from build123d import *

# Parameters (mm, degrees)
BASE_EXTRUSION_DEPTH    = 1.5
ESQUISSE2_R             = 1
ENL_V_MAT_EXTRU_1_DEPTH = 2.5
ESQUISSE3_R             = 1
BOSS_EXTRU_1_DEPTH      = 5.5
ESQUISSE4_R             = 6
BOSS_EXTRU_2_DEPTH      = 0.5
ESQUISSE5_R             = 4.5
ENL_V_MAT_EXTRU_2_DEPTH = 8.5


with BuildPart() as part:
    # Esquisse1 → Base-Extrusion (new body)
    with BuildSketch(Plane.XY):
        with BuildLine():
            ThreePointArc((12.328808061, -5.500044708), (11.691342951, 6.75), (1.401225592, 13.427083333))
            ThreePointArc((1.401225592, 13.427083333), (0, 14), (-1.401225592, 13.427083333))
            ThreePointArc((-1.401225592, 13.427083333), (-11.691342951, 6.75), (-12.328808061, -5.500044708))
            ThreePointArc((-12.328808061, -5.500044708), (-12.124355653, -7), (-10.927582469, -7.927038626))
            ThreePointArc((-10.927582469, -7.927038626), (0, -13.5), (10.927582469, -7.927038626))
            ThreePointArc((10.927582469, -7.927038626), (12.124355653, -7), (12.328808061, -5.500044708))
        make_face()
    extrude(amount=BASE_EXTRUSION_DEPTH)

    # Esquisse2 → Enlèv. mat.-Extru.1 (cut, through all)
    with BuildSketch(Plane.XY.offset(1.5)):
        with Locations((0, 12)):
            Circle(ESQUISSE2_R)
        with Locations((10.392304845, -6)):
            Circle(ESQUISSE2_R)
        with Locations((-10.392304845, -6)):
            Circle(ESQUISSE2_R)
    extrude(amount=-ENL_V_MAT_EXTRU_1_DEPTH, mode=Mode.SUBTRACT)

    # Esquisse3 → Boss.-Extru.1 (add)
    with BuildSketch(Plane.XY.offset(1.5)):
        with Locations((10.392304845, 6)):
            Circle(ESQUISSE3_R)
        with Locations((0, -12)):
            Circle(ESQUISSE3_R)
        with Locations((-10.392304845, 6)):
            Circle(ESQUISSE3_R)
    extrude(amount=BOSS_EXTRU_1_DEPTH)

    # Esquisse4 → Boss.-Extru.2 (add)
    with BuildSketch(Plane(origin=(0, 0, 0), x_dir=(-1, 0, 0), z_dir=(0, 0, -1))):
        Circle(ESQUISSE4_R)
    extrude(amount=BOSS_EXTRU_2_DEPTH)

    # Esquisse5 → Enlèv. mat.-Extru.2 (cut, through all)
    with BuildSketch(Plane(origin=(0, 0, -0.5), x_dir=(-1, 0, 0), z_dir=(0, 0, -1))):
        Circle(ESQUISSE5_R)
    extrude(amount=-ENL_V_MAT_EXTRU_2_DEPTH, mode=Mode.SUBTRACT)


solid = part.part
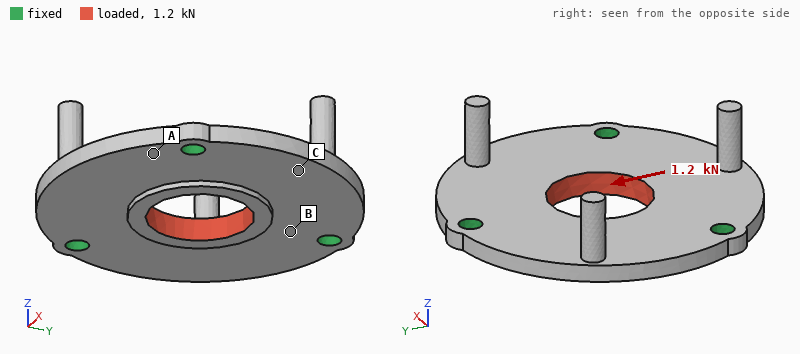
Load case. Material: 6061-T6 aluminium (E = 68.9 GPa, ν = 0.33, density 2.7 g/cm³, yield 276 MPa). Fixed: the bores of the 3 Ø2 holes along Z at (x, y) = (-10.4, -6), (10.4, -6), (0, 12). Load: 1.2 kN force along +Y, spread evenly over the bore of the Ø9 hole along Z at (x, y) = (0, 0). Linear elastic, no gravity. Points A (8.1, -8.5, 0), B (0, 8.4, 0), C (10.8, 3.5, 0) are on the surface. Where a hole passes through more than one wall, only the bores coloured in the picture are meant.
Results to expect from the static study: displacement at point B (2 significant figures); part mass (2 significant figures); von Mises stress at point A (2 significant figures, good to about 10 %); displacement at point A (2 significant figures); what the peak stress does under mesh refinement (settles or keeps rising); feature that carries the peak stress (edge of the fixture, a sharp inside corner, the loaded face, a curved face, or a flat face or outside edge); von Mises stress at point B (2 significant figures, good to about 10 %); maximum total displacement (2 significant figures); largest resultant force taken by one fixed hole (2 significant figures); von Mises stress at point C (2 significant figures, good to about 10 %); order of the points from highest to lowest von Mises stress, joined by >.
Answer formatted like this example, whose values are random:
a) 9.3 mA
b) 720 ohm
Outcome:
a) 2.2 µm
b) 2.2 g
c) 35 MPa
d) 3.2 µm
e) keeps rising
f) edge of the fixture
g) 55 MPa
h) 11 µm
i) 410 N
j) 15 MPa
k) B > A > C
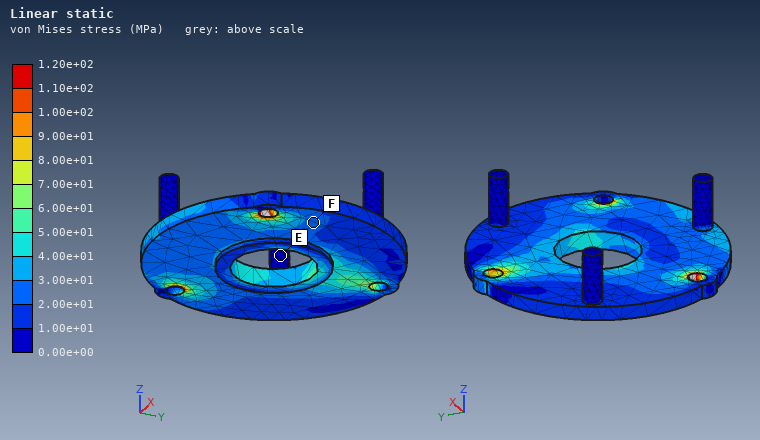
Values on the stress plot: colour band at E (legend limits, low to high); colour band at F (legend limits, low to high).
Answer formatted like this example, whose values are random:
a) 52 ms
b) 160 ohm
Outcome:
a) 0.00e+00 to 1.00e+01 MPa
b) 2.00e+01 to 3.00e+01 MPa
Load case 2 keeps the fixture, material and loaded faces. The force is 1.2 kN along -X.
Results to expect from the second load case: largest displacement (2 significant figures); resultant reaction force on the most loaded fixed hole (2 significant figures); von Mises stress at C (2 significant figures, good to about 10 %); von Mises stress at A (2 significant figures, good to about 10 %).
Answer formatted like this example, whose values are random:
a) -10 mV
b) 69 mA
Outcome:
a) 9.5 µm
b) 410 N
c) 19 MPa
d) 20 MPa
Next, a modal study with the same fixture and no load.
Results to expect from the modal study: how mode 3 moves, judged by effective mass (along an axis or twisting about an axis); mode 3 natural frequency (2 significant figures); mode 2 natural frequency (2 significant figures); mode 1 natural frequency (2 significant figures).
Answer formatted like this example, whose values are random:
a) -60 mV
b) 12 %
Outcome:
a) along Z
b) 14 kHz
c) 12 kHz
d) 12 kHz
